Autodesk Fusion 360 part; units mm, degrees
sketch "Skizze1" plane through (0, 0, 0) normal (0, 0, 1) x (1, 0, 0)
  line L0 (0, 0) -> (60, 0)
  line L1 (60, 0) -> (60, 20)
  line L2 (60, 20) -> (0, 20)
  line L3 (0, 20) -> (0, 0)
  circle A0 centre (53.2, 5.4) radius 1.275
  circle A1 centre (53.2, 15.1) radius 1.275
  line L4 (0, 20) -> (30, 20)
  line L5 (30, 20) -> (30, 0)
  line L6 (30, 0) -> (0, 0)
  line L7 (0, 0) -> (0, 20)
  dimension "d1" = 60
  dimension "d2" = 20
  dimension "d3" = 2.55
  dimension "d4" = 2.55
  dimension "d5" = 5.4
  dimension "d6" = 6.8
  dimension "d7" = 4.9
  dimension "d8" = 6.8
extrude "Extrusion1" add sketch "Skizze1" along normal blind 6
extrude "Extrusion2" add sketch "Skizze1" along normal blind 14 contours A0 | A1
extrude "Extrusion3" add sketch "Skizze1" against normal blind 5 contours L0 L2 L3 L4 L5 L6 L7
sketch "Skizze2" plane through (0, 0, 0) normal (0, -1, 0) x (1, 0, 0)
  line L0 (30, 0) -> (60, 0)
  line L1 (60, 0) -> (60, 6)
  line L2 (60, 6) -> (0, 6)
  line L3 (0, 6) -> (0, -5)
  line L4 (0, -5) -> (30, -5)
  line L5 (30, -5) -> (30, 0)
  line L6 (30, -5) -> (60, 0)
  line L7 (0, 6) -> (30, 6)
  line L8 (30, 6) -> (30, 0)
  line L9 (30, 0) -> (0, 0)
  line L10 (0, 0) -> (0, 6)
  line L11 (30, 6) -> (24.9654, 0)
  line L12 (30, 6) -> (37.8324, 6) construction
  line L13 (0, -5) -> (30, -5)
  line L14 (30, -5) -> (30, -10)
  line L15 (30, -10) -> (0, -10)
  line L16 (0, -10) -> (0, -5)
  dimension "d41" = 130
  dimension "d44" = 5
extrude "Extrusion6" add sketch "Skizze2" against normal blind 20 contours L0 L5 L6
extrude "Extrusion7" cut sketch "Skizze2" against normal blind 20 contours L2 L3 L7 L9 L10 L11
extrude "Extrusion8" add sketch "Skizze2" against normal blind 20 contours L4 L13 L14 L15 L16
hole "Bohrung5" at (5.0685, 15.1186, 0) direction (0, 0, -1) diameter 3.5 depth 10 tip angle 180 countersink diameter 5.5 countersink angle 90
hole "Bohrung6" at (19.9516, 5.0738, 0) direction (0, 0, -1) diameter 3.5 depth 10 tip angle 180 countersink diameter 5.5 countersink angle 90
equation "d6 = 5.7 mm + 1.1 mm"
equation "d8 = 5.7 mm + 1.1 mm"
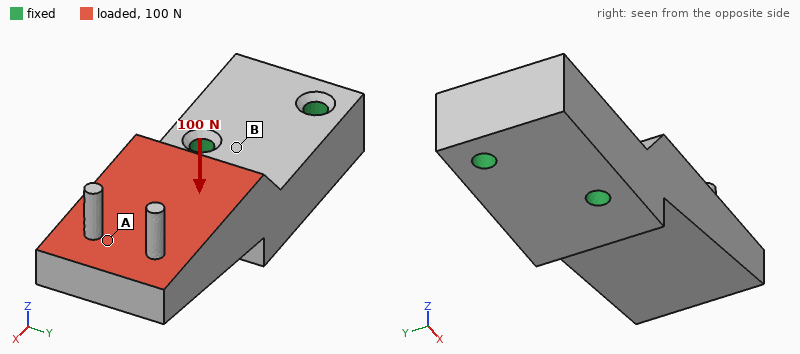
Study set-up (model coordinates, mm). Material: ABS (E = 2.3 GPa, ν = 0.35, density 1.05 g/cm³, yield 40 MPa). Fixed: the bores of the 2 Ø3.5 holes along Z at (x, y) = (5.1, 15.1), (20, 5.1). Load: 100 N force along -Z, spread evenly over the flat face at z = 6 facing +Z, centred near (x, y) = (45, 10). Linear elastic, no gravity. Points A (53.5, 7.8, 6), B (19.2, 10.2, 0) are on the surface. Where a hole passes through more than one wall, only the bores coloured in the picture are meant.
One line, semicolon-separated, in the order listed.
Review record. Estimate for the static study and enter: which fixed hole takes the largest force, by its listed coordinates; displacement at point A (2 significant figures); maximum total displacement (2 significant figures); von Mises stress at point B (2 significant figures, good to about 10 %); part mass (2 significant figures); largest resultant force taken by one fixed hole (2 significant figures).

(20, 5.1); 0.39 mm; 0.50 mm; 4.4 MPa; 12 g; 140 N
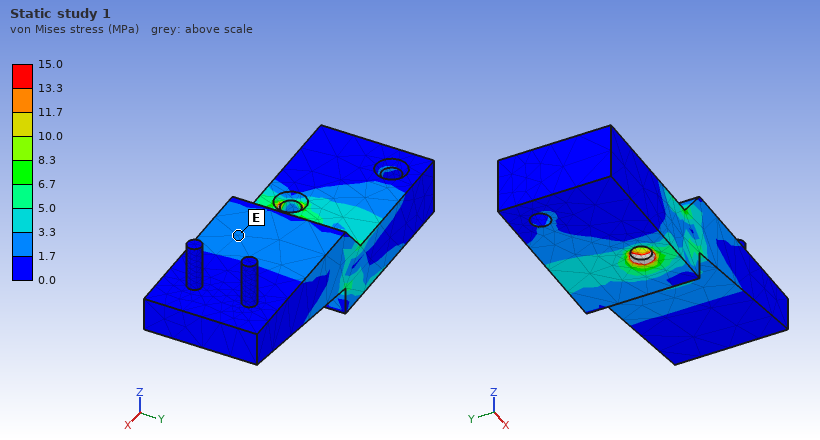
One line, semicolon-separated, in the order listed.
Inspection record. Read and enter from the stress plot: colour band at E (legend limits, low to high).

1.7 to 3.3 MPa
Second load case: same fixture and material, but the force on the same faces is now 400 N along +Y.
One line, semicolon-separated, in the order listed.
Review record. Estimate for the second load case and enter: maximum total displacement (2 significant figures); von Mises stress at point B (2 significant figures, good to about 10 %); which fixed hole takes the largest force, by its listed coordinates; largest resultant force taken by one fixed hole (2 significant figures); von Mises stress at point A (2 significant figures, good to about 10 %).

0.74 mm; 8.6 MPa; (20, 5.1); 800 N; 3.5 MPa
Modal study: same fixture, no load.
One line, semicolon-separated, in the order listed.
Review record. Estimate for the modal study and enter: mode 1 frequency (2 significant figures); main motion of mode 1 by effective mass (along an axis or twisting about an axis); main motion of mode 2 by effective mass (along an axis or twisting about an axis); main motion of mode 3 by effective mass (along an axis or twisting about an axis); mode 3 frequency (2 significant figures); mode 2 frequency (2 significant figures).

1200 Hz; along Z; along Y; twisting about X; 3900 Hz; 2100 Hz
